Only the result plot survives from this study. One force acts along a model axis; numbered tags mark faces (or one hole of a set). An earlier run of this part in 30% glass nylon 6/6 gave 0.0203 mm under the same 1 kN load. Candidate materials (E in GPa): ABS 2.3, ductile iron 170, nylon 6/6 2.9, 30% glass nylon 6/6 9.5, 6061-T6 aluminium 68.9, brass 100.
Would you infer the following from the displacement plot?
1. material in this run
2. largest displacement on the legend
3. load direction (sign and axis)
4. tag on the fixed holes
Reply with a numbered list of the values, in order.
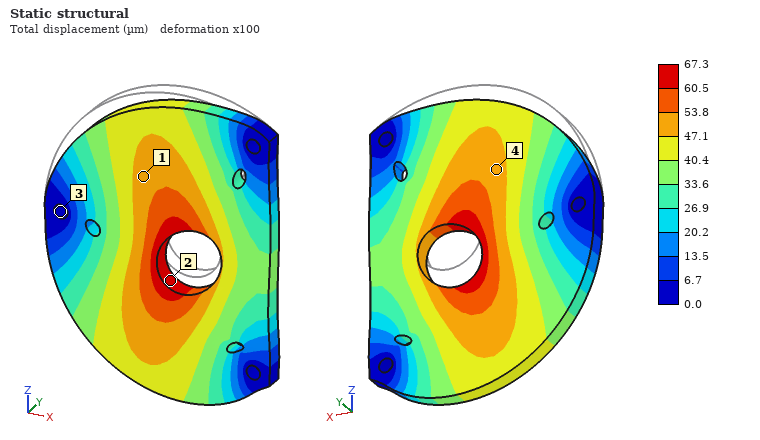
1. nylon 6/6
2. 67.3 µm
3. -Z
4. 3
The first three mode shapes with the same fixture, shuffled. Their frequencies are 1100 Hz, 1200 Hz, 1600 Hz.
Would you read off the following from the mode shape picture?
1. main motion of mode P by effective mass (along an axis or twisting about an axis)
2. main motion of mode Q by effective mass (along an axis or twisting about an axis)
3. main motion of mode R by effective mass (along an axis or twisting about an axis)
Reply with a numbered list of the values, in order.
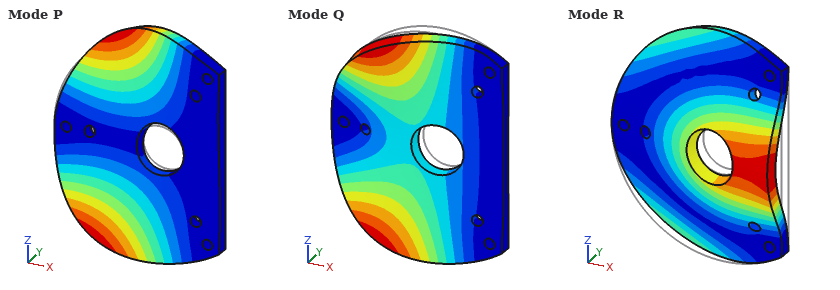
1. twisting about X
2. along Y
3. along Y
